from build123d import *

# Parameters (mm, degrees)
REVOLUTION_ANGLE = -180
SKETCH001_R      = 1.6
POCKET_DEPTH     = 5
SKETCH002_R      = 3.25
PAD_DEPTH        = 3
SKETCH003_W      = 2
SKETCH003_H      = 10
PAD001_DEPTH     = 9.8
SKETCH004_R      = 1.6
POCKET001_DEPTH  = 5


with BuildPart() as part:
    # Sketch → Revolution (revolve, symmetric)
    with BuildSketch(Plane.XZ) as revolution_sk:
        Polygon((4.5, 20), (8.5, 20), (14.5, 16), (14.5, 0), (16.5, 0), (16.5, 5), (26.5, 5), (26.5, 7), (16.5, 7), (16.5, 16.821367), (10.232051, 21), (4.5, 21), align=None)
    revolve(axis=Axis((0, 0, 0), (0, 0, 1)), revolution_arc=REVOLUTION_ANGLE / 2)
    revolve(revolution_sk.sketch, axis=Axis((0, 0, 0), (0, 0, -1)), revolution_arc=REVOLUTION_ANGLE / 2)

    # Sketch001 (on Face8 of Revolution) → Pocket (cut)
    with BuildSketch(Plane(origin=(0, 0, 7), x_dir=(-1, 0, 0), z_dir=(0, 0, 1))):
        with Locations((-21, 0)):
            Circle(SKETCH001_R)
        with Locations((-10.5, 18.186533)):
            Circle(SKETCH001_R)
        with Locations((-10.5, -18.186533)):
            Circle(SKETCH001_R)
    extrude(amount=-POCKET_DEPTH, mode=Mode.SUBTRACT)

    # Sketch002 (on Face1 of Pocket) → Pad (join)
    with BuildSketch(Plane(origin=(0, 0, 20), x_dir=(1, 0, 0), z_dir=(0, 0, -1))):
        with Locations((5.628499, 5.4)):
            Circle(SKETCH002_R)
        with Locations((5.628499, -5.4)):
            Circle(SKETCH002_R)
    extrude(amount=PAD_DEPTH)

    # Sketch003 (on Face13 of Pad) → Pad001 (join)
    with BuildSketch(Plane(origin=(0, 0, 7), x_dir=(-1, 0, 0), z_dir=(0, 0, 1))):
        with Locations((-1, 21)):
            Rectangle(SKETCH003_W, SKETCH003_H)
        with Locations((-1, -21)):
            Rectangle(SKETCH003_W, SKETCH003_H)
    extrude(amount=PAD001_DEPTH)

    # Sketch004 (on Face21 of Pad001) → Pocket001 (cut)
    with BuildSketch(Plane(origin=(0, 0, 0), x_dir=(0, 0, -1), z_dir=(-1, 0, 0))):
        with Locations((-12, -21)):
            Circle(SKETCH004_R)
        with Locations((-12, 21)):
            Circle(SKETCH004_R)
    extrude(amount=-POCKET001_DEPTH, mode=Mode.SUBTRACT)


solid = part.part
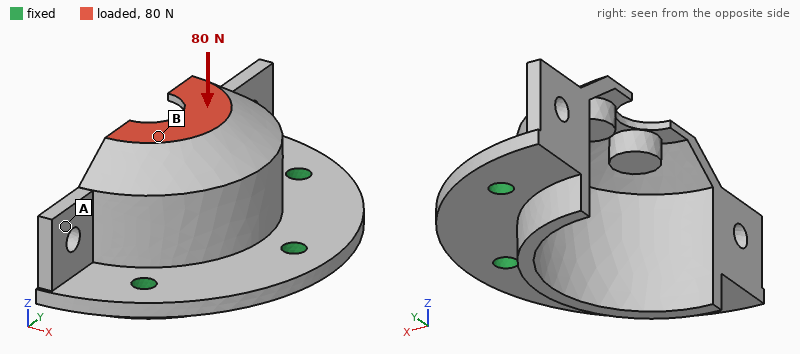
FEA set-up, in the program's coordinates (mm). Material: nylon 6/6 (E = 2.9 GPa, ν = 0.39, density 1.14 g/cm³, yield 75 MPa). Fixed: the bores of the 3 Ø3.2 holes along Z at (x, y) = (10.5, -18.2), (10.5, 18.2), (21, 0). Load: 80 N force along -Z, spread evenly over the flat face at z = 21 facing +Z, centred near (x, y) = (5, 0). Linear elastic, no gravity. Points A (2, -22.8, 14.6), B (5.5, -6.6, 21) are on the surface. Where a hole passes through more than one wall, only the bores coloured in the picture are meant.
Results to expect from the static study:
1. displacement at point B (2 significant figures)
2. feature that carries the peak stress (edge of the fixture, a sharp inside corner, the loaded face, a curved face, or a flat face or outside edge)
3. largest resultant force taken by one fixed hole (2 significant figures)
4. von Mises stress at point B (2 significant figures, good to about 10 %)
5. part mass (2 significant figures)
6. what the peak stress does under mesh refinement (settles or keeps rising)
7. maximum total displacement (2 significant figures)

0.20 mm
edge of the fixture
55 N
7.7 MPa
4.6 g
keeps rising
0.35 mm
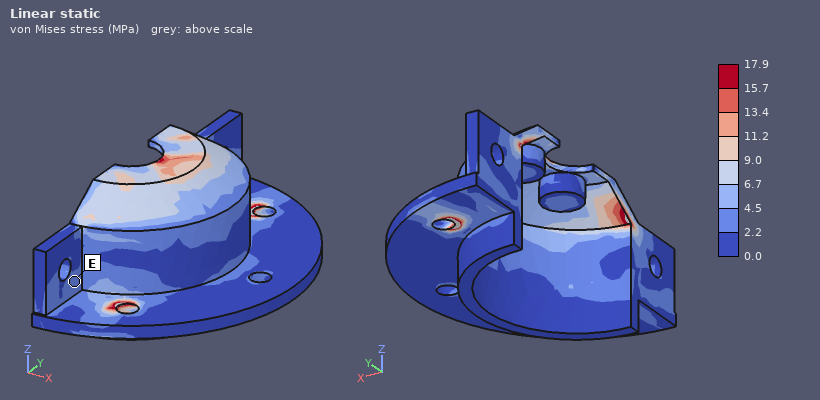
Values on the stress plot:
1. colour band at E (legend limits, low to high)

2.2 to 4.5 MPa
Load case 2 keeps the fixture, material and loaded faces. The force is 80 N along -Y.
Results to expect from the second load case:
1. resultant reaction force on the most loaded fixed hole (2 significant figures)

45 N
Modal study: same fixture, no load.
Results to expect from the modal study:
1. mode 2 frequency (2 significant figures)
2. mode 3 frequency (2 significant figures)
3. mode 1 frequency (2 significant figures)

2400 Hz
4400 Hz
2200 Hz
